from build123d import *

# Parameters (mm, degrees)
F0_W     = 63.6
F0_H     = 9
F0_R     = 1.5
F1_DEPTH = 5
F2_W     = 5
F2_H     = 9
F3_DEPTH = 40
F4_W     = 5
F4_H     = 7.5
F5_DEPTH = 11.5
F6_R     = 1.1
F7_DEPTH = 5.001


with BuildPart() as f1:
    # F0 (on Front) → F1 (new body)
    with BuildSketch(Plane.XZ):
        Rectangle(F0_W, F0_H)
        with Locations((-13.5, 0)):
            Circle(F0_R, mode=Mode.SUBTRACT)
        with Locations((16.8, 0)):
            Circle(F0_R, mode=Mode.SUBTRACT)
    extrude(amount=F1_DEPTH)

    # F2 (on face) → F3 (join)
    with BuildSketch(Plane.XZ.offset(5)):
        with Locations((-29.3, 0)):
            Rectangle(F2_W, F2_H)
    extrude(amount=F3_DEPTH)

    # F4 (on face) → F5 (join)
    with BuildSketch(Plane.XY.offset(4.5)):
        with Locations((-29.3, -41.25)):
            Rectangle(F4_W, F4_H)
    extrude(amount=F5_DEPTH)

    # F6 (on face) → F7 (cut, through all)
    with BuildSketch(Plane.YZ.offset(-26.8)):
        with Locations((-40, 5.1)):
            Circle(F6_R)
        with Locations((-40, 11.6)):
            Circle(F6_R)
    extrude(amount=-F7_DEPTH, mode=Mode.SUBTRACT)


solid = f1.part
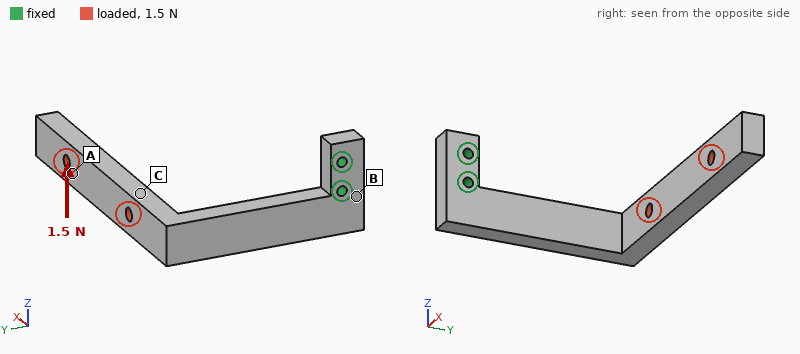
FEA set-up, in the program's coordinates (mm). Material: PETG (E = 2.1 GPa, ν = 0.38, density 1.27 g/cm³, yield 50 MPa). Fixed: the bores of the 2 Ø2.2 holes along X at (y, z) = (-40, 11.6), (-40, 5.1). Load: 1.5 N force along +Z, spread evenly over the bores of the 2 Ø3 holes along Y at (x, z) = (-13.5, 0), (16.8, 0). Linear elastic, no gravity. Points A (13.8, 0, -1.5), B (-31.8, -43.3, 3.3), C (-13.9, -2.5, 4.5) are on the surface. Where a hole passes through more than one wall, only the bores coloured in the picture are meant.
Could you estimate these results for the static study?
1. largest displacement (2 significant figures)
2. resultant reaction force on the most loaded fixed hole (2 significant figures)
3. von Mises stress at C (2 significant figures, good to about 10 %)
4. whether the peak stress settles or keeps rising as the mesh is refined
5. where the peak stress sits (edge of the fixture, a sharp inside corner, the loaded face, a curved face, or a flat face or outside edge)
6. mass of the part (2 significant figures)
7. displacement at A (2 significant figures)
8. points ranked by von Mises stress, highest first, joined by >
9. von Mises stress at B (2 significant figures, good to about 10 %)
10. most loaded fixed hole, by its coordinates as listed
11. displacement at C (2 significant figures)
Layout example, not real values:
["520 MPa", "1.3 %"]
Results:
["0.74 mm", "6.5 N", "0.35 MPa", "keeps rising", "edge of the fixture", "6.3 g", "0.54 mm", "B > C > A", "1.2 MPa", "(-40, 5.1)", "0.24 mm"]
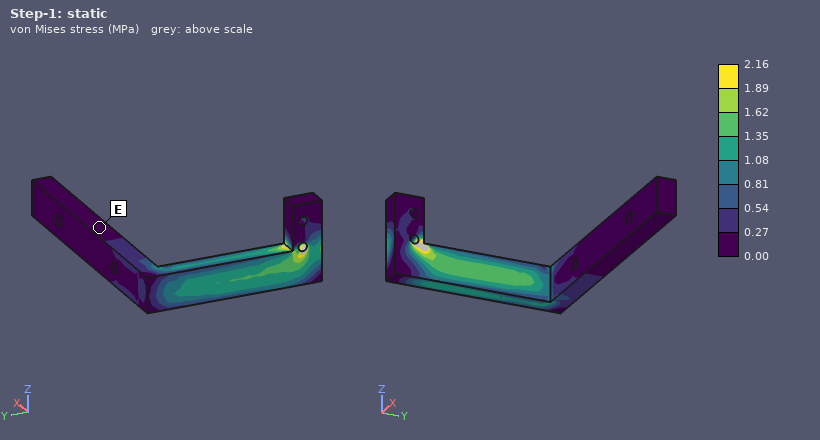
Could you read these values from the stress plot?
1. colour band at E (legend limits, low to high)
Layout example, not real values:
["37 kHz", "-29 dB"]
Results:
["0.00 to 0.27 MPa"]
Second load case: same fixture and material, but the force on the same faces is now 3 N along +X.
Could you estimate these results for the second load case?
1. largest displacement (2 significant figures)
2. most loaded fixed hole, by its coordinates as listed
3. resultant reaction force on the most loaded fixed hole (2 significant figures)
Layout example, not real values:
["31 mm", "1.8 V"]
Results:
["0.84 mm", "(-40, 5.1)", "3.2 N"]
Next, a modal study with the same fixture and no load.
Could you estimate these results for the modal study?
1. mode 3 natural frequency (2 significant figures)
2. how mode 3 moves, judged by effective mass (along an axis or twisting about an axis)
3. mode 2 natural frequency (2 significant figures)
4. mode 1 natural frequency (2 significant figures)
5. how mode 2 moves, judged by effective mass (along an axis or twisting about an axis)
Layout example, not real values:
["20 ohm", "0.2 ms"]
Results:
["390 Hz", "along X", "150 Hz", "130 Hz", "along Z"]
